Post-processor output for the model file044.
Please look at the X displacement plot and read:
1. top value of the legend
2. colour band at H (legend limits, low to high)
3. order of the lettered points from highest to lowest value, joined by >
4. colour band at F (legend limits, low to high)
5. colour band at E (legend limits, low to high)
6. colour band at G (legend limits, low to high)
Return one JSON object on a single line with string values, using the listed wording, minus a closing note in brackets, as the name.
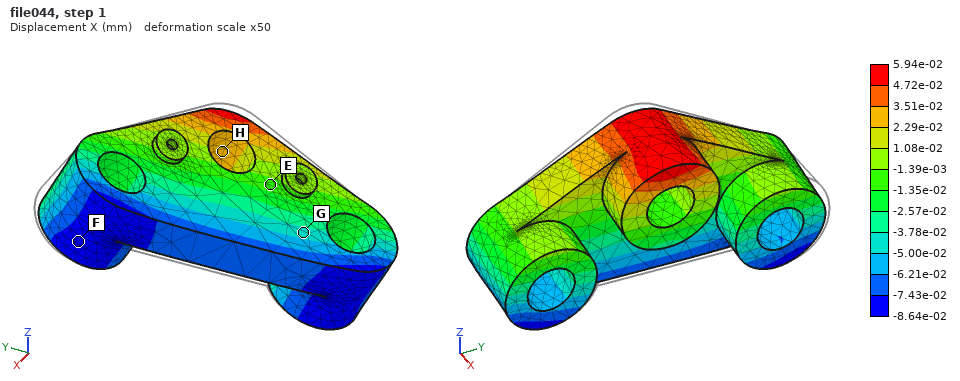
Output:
{"top value of the legend": "5.94e-02 mm", "colour band at H": "2.29e-02 to 3.51e-02 mm", "order of the lettered points from highest to lowest value, joined by >": "H > E > G > F", "colour band at F": "-8.64e-02 to -7.43e-02 mm", "colour band at E": "-1.35e-02 to -1.39e-03 mm", "colour band at G": "-5.00e-02 to -3.78e-02 mm"}
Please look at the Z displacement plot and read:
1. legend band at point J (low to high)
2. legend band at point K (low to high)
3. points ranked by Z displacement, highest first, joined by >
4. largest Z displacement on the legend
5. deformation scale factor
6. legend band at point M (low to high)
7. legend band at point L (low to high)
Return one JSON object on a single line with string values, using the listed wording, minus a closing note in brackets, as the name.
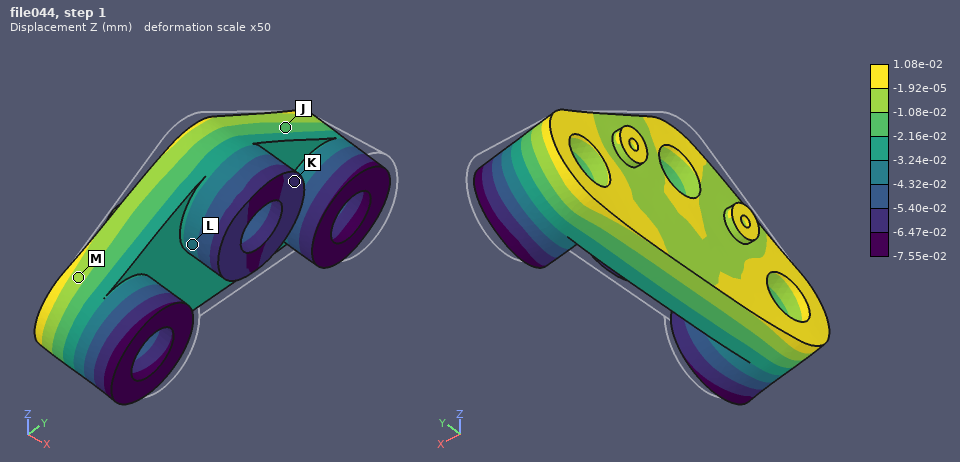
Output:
{"legend band at point J": "-2.16e-02 to -1.08e-02 mm", "legend band at point K": "-6.47e-02 to -5.40e-02 mm", "points ranked by Z displacement, highest first, joined by >": "M > J > L > K", "largest Z displacement on the legend": "1.08e-02 mm", "deformation scale factor": "50", "legend band at point M": "-1.08e-02 to -1.92e-05 mm", "legend band at point L": "-4.32e-02 to -3.24e-02 mm"}
